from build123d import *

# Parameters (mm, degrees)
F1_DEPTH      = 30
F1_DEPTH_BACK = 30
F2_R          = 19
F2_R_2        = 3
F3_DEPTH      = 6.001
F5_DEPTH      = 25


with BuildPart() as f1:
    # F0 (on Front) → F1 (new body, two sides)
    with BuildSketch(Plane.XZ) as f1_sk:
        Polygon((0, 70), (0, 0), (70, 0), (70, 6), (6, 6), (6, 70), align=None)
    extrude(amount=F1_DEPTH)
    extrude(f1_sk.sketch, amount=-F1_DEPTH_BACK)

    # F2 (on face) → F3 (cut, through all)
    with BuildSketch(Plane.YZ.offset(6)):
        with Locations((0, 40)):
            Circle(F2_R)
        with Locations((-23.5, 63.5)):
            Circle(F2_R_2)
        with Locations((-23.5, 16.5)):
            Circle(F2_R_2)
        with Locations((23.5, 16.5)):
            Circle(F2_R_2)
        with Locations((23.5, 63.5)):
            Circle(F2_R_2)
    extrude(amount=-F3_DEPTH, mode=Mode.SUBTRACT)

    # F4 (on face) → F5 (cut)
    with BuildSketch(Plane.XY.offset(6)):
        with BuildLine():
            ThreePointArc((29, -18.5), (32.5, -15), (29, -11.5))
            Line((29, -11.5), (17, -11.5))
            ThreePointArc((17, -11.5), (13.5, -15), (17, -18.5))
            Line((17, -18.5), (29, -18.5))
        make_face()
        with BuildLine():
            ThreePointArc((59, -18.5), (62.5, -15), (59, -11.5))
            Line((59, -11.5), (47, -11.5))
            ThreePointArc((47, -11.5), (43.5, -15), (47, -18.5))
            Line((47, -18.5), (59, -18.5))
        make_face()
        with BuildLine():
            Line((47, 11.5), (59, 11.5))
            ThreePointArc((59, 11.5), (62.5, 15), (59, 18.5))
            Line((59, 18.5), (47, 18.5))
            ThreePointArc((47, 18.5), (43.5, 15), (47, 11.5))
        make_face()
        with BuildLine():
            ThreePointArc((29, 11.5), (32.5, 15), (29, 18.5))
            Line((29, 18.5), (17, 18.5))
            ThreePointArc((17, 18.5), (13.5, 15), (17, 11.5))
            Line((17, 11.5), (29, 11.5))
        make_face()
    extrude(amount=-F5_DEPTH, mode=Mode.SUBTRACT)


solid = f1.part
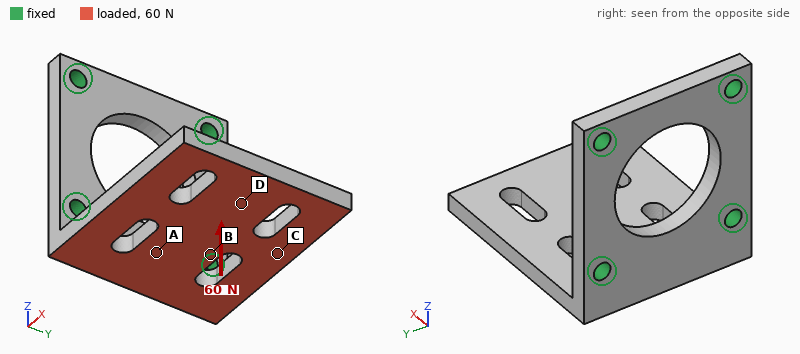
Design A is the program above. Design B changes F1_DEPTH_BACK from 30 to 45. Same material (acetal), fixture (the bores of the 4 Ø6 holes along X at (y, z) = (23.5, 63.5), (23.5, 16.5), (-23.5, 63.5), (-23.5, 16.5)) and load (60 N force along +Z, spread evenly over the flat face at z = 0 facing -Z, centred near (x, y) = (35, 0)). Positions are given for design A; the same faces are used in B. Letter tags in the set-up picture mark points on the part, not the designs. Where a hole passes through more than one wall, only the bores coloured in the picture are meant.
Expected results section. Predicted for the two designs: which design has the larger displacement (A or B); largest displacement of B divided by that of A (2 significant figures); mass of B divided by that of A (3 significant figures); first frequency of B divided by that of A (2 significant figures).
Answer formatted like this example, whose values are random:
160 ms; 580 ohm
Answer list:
A; 0.80; 1.32; 0.99
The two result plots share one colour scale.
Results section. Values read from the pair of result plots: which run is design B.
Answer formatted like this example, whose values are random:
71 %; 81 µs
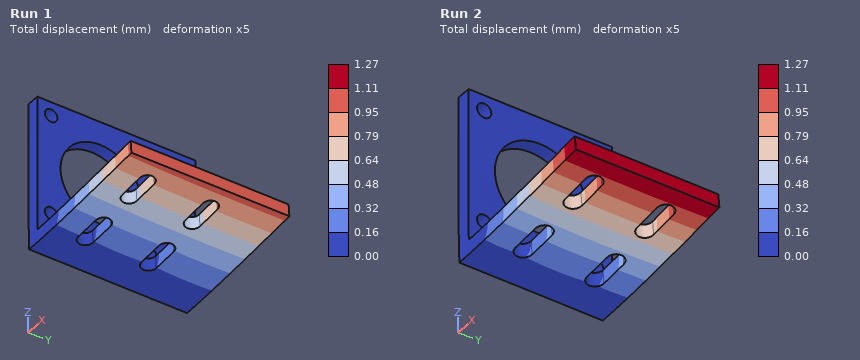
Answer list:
Run 1
